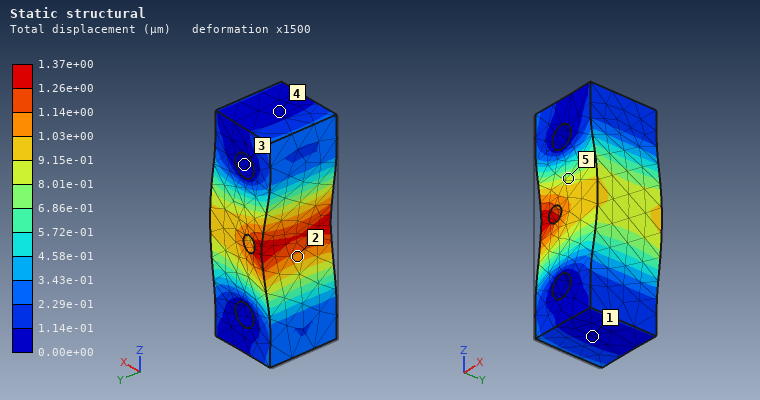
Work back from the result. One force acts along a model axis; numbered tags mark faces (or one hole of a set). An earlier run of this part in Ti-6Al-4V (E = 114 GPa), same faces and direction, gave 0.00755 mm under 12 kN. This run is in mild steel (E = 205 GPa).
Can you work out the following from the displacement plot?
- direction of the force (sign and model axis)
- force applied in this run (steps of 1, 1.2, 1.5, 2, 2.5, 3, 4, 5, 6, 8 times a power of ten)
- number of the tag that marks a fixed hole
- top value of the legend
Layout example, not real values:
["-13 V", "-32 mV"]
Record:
["+X", "4 kN", "3", "1.37e+00 µm"]
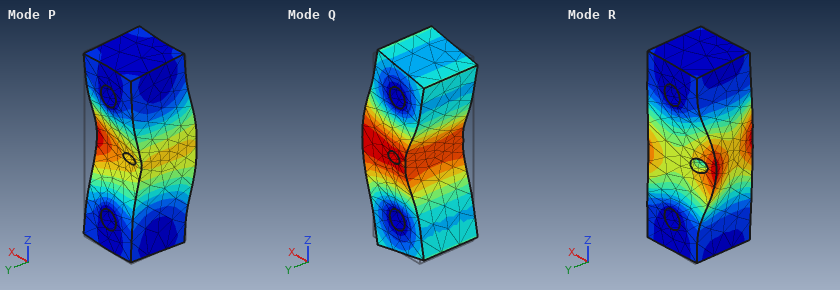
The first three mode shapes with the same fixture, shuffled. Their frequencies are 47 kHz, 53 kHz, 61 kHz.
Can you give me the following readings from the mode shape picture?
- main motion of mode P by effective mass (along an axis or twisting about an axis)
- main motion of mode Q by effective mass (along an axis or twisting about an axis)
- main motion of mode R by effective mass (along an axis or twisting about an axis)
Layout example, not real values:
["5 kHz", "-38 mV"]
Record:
["along Y", "along X", "twisting about Z"]
